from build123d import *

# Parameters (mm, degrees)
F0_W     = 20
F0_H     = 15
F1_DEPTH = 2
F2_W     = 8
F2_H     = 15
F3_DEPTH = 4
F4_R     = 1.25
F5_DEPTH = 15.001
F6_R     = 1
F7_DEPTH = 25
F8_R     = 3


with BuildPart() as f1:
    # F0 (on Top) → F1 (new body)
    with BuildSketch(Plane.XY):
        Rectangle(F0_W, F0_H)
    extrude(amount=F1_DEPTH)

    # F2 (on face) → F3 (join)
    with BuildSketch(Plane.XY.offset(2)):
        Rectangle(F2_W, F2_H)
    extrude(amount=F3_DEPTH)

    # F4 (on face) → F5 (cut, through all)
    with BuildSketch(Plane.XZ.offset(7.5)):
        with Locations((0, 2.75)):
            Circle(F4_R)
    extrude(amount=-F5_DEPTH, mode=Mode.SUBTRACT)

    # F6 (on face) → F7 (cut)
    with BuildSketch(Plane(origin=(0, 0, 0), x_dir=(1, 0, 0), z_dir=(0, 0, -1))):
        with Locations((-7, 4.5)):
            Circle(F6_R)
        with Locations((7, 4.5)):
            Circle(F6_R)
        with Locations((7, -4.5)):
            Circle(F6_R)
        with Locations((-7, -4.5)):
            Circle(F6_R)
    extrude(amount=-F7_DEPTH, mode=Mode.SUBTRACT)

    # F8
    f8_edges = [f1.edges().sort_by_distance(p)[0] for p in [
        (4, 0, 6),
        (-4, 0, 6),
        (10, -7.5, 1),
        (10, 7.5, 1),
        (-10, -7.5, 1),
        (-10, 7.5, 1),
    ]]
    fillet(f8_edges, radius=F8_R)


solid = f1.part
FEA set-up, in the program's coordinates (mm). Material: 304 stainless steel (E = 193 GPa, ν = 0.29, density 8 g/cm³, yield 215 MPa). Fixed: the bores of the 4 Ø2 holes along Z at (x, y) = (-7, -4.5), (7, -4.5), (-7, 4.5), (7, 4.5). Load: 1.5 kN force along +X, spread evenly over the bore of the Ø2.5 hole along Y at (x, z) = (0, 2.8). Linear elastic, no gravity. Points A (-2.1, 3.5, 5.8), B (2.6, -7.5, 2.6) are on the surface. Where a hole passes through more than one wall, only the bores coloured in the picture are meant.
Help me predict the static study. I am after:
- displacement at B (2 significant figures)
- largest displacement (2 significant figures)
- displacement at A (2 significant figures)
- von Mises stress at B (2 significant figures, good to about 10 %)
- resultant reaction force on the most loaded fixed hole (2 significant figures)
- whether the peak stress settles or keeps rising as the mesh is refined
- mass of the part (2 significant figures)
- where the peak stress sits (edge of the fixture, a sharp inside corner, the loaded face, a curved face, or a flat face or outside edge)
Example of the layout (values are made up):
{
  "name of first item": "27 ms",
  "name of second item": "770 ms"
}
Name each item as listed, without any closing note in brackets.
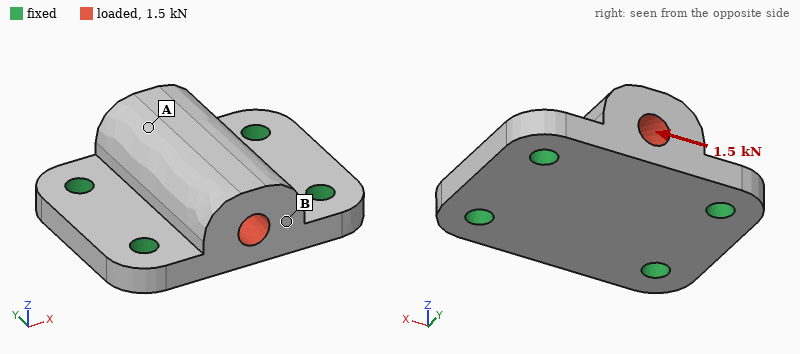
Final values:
{
  "displacement at B": "0.95 µm",
  "largest displacement": "1.7 µm",
  "displacement at A": "1.7 µm",
  "von Mises stress at B": "24 MPa",
  "resultant reaction force on the most loaded fixed hole": "400 N",
  "whether the peak stress settles or keeps rising as the mesh is refined": "keeps rising",
  "mass of the part": "7.3 g",
  "where the peak stress sits": "edge of the fixture"
}
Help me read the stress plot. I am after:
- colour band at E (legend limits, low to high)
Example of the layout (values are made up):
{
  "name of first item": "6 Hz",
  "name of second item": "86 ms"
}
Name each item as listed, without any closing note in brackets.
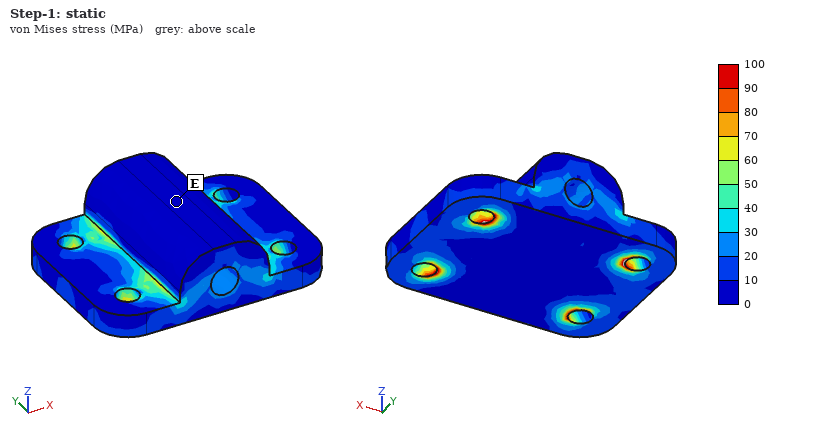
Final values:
{
  "colour band at E": "0 to 10 MPa"
}
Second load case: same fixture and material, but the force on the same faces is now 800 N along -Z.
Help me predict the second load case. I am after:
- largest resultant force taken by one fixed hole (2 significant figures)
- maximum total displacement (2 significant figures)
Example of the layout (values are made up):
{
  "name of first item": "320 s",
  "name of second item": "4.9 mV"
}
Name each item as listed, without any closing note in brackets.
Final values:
{
  "largest resultant force taken by one fixed hole": "210 N",
  "maximum total displacement": "2.4 µm"
}
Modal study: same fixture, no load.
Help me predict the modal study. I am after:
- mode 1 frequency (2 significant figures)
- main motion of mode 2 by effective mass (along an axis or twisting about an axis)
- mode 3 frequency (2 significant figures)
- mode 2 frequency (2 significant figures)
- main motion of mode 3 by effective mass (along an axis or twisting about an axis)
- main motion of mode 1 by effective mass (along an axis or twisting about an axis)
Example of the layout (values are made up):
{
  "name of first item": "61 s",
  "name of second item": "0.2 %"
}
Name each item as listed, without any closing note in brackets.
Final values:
{
  "mode 1 frequency": "43 kHz",
  "main motion of mode 2 by effective mass": "along Z",
  "mode 3 frequency": "69 kHz",
  "mode 2 frequency": "46 kHz",
  "main motion of mode 3 by effective mass": "along X",
  "main motion of mode 1 by effective mass": "along Y"
}
